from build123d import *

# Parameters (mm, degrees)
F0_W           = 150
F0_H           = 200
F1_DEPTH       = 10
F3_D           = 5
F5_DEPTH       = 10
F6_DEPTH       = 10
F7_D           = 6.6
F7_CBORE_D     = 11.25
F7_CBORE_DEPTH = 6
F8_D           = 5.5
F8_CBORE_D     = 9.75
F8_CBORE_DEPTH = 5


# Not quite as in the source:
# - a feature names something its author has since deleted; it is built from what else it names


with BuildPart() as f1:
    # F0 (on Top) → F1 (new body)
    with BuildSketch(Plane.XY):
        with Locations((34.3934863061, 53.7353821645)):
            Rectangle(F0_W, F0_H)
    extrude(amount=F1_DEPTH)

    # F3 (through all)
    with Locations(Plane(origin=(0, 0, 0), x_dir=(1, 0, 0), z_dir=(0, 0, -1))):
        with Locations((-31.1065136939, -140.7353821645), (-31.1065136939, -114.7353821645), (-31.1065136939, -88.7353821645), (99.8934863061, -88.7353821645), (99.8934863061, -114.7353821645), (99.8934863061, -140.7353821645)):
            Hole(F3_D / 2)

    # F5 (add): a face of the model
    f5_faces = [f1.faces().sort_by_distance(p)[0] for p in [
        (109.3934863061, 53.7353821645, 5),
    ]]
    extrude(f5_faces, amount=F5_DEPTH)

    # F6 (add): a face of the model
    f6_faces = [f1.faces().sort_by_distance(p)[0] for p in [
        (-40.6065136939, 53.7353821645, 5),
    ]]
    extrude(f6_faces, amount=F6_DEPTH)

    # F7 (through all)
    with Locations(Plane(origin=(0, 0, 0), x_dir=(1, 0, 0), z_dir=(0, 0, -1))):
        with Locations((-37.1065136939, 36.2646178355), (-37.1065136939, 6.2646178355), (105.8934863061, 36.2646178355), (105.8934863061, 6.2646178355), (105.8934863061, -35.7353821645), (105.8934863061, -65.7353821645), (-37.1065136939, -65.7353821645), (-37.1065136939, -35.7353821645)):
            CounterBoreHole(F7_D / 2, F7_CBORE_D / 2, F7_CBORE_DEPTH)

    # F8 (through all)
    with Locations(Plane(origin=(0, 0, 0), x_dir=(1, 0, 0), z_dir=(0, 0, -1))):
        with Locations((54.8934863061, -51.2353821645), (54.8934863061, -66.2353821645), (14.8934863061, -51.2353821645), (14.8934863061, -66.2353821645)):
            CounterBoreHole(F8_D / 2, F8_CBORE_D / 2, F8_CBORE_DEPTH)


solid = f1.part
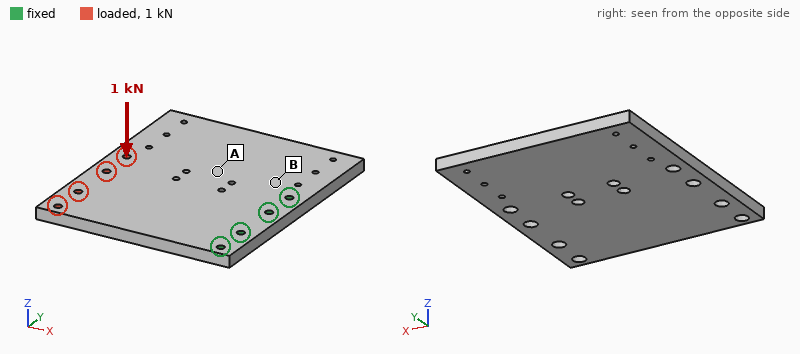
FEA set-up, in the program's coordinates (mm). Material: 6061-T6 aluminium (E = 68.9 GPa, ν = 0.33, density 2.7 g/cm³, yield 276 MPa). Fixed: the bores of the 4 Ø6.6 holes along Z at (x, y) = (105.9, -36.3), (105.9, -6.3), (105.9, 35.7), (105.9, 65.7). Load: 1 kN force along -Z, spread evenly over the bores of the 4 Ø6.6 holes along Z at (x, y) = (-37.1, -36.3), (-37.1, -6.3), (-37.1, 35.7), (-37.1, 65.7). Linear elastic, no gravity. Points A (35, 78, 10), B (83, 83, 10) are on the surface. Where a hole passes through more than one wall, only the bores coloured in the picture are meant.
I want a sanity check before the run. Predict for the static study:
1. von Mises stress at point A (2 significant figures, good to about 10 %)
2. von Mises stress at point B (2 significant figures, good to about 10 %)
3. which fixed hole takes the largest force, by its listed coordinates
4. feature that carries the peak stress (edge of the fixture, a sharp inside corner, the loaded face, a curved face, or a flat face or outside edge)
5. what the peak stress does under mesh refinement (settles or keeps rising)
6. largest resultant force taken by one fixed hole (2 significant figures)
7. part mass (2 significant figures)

19 MPa
30 MPa
(105.9, 35.7)
edge of the fixture
keeps rising
780 N
890 g
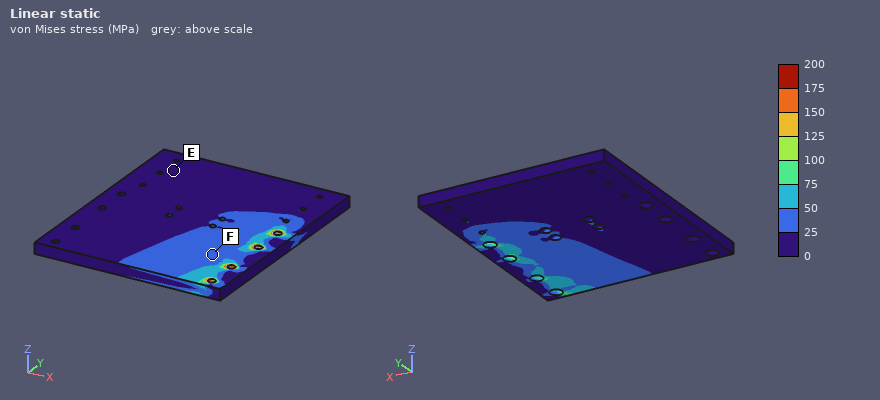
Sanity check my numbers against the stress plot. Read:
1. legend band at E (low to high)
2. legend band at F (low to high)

0 to 25 MPa
25 to 50 MPa
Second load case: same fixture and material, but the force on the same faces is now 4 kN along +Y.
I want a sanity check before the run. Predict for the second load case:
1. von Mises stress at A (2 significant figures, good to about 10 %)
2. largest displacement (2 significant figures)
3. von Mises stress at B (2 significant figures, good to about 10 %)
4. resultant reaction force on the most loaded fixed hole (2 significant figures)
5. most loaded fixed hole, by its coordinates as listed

7.7 MPa
0.26 mm
10.0 MPa
5.3 kN
(105.9, 65.7)
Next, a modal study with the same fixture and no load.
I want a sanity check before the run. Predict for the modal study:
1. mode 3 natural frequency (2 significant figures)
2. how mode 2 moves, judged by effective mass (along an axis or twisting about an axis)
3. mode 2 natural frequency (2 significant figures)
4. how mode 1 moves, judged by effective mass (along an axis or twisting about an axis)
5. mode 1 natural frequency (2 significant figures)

1100 Hz
twisting about X
480 Hz
along Z
220 Hz
